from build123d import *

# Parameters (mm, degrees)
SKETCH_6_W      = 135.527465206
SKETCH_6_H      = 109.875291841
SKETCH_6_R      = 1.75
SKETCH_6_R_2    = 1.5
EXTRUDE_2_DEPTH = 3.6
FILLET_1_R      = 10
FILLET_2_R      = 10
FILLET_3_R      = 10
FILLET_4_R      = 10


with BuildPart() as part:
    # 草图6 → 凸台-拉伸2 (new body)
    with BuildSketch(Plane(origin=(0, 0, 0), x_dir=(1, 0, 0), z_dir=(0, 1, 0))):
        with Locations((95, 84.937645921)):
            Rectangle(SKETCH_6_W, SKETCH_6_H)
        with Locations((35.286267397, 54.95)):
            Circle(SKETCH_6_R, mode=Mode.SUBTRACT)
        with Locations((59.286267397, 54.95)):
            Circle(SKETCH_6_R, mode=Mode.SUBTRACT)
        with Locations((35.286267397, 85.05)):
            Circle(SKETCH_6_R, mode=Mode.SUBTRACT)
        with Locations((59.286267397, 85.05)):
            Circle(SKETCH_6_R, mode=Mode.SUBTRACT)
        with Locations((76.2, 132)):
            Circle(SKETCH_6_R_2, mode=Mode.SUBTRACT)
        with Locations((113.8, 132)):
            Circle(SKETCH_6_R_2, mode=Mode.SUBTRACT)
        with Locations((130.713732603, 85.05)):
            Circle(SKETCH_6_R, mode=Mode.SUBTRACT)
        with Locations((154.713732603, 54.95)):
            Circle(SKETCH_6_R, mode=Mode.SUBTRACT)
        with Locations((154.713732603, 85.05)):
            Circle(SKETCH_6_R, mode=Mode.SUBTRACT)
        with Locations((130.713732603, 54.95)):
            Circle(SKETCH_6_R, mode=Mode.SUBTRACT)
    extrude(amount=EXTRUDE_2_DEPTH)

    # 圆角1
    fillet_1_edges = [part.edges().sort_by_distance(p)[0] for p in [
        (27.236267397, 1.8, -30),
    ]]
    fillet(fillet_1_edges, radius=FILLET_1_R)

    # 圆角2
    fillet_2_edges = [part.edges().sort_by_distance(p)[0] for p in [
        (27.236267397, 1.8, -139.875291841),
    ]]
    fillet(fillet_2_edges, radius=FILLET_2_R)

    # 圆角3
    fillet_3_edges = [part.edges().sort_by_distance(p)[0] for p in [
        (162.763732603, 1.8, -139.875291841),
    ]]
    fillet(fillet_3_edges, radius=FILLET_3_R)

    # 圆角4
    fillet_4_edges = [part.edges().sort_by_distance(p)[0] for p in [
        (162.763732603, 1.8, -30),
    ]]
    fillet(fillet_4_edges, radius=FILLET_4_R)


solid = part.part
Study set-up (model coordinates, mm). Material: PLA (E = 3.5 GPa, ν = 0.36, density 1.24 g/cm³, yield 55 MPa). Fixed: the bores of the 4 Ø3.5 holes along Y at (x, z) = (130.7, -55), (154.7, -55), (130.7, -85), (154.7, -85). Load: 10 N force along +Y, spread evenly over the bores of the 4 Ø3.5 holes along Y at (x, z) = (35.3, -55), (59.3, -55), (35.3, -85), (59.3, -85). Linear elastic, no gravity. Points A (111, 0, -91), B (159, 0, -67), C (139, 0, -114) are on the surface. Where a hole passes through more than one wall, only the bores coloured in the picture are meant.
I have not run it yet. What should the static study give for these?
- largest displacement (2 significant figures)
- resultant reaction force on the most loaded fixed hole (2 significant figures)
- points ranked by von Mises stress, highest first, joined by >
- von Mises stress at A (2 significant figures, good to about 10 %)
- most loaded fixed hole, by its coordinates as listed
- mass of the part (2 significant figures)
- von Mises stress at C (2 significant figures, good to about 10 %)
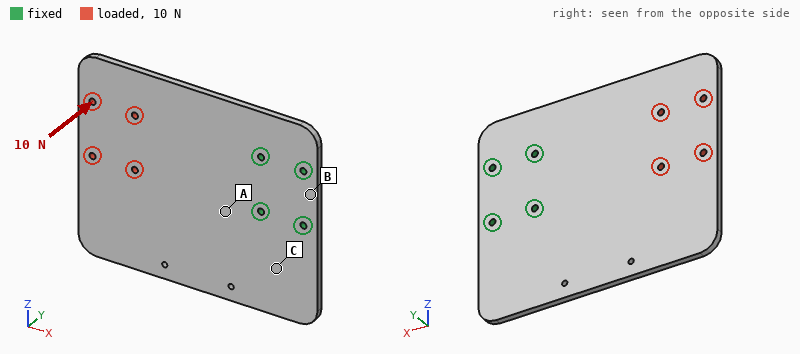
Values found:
2.1 mm
17 N
A > C > B
2.5 MPa
(130.7, -85)
66 g
1.3 MPa
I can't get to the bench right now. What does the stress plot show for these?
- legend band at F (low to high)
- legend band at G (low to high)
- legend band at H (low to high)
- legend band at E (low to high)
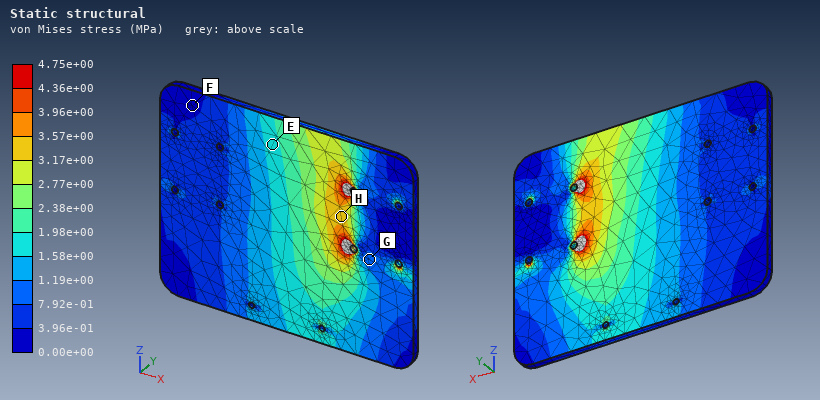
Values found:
0.00e+00 to 3.96e-01 MPa
7.92e-01 to 1.19e+00 MPa
3.17e+00 to 3.57e+00 MPa
1.58e+00 to 1.98e+00 MPa
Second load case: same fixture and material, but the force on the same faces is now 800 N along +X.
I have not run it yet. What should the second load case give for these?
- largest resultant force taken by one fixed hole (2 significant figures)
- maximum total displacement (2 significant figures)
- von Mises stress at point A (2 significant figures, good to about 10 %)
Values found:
300 N
97 µm
2.8 MPa
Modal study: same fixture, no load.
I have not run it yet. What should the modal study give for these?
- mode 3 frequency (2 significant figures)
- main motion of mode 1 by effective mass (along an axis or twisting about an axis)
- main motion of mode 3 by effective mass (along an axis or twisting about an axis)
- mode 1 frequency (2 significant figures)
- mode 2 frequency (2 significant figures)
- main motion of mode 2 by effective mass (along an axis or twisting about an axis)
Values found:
360 Hz
along Y
along Y
86 Hz
170 Hz
twisting about X
